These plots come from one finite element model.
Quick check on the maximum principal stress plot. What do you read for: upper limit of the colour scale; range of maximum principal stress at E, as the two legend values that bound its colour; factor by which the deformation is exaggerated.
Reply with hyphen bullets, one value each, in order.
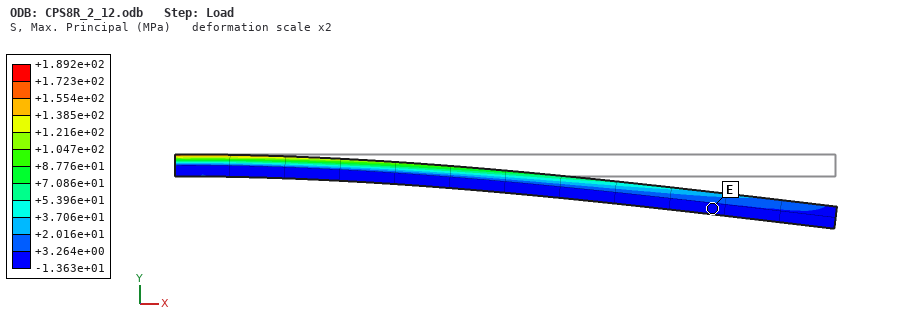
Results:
- +1.892e+02 MPa
- -1.363e+01 to +3.264e+00 MPa
- 2
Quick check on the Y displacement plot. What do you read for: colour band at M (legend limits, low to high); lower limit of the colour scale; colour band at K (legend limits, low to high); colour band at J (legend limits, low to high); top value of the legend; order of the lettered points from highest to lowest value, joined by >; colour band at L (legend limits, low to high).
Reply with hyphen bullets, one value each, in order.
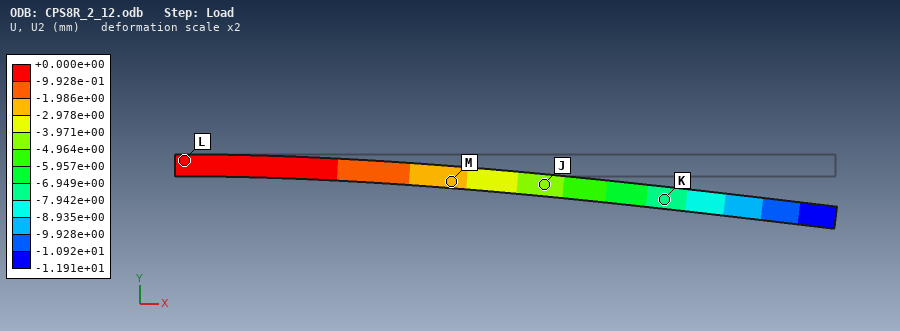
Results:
- -2.978e+00 to -1.986e+00 mm
- -1.191e+01 mm
- -7.942e+00 to -6.949e+00 mm
- -4.964e+00 to -3.971e+00 mm
- +0.000e+00 mm
- L > M > J > K
- -9.928e-01 to +0.000e+00 mm
